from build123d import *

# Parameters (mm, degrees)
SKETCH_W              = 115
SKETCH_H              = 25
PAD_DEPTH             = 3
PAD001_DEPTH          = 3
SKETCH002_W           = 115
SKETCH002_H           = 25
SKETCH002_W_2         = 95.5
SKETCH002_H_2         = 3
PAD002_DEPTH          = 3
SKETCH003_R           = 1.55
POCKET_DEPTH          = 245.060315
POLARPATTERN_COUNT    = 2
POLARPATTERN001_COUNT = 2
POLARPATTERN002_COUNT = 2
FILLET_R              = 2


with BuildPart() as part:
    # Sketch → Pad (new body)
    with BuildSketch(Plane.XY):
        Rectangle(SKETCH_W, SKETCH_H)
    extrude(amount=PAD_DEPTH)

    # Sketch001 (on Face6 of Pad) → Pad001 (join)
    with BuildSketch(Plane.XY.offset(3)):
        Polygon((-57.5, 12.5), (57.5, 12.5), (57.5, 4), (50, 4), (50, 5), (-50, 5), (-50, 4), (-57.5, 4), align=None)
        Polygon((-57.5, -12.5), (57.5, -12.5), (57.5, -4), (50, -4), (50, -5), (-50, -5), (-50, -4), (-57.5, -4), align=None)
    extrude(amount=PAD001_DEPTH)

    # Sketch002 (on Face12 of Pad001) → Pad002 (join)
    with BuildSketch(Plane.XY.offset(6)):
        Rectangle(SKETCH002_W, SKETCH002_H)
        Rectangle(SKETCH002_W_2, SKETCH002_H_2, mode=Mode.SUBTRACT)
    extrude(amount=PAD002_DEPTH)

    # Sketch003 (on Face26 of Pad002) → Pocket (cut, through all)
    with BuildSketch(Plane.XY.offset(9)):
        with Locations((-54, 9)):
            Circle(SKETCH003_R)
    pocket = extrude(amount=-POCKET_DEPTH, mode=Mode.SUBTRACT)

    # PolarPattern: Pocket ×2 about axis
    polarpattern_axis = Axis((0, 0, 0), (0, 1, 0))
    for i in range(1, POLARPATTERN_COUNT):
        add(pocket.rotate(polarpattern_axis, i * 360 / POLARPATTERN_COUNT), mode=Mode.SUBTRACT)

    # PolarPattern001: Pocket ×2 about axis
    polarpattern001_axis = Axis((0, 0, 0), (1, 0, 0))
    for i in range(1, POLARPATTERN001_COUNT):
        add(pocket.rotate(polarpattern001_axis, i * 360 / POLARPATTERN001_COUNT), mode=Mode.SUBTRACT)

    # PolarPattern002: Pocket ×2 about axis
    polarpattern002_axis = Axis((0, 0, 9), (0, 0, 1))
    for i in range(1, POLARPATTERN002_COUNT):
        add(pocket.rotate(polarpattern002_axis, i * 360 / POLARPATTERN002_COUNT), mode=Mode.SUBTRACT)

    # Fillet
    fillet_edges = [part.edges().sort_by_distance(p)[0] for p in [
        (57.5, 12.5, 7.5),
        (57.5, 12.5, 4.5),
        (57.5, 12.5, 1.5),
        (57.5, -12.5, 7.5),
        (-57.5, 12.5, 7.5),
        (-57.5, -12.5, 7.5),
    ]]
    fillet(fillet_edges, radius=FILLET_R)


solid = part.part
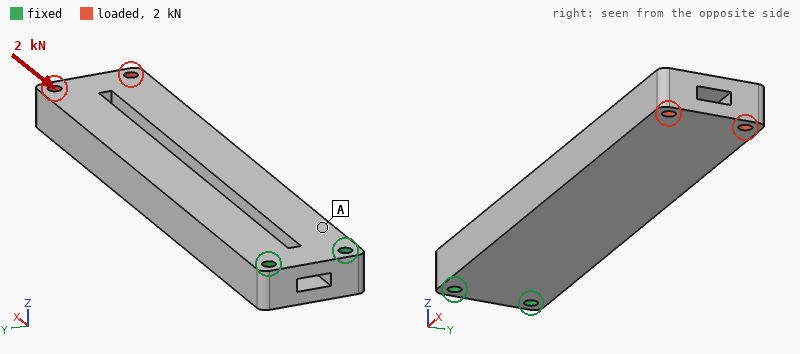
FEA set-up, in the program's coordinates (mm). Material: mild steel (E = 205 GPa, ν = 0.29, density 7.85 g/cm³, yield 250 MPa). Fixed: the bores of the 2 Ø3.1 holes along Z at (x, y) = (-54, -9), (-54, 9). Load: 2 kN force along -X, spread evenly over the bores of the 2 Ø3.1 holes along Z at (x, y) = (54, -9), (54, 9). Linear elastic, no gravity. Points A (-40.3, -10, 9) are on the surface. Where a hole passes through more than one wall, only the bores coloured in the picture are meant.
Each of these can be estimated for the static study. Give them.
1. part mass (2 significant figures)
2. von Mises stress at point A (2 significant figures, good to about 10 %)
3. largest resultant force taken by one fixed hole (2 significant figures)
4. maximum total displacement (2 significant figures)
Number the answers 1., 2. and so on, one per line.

1. 170 g
2. 12 MPa
3. 1.0 kN
4. 8.6 µm
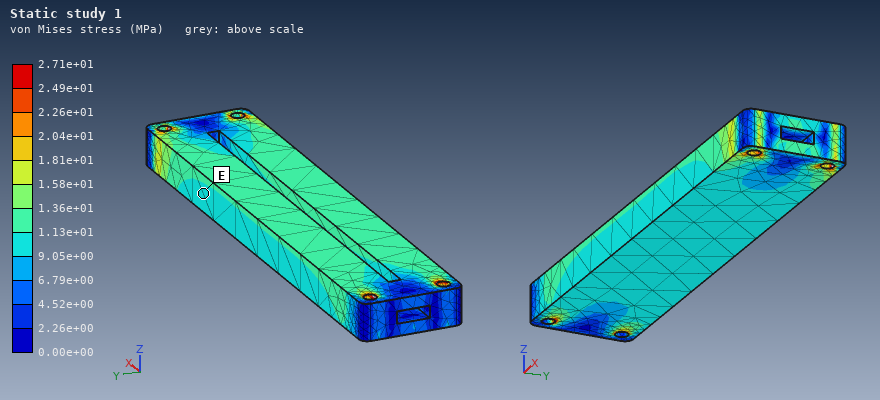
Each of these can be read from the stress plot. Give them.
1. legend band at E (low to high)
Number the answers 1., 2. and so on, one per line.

1. 9.05e+00 to 1.13e+01 MPa
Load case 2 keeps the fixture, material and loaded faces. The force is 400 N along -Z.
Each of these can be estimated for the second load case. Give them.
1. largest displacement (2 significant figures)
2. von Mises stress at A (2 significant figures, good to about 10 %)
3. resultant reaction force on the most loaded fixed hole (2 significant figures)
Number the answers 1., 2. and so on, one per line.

1. 0.64 mm
2. 130 MPa
3. 230 N
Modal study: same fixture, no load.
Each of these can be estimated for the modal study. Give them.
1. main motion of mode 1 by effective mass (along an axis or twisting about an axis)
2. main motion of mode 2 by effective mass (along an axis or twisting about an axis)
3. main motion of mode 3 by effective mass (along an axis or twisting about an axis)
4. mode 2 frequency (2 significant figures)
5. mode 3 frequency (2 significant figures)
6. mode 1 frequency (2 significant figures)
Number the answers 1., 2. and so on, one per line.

1. along Z
2. along Y
3. twisting about X
4. 1600 Hz
5. 3100 Hz
6. 620 Hz
